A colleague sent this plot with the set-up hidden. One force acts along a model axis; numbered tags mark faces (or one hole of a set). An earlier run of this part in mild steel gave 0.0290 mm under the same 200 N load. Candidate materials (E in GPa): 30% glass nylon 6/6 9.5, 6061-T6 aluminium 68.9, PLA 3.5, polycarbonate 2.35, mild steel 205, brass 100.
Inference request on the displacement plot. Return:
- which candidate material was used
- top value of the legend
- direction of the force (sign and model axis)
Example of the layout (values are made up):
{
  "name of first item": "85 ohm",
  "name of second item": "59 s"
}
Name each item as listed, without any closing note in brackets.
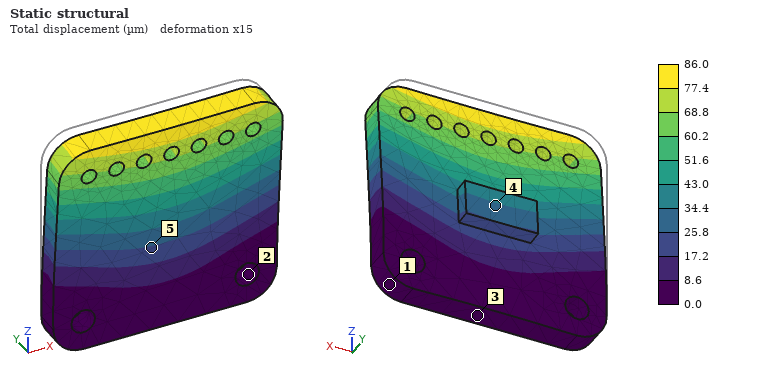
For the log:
{
  "which candidate material was used": "6061-T6 aluminium",
  "top value of the legend": "86.0 µm",
  "direction of the force": "-Y"
}
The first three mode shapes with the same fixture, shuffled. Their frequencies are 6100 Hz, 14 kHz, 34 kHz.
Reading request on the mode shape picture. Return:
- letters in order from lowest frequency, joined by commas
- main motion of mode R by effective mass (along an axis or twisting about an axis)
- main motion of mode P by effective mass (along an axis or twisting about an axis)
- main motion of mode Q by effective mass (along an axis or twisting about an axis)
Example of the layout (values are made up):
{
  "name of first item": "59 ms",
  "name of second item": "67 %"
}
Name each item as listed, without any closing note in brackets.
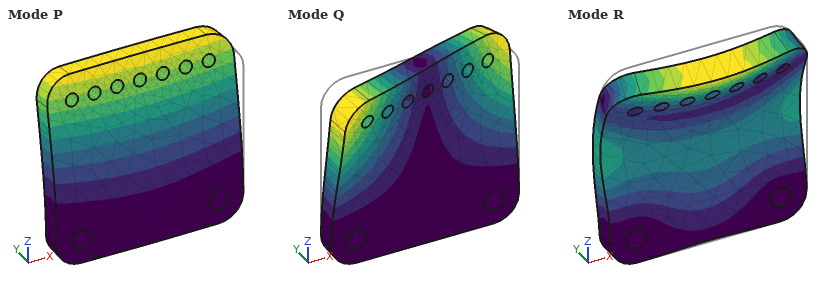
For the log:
{
  "letters in order from lowest frequency, joined by commas": "P, Q, R",
  "main motion of mode R by effective mass": "along Y",
  "main motion of mode P by effective mass": "along Y",
  "main motion of mode Q by effective mass": "twisting about Z"
}
